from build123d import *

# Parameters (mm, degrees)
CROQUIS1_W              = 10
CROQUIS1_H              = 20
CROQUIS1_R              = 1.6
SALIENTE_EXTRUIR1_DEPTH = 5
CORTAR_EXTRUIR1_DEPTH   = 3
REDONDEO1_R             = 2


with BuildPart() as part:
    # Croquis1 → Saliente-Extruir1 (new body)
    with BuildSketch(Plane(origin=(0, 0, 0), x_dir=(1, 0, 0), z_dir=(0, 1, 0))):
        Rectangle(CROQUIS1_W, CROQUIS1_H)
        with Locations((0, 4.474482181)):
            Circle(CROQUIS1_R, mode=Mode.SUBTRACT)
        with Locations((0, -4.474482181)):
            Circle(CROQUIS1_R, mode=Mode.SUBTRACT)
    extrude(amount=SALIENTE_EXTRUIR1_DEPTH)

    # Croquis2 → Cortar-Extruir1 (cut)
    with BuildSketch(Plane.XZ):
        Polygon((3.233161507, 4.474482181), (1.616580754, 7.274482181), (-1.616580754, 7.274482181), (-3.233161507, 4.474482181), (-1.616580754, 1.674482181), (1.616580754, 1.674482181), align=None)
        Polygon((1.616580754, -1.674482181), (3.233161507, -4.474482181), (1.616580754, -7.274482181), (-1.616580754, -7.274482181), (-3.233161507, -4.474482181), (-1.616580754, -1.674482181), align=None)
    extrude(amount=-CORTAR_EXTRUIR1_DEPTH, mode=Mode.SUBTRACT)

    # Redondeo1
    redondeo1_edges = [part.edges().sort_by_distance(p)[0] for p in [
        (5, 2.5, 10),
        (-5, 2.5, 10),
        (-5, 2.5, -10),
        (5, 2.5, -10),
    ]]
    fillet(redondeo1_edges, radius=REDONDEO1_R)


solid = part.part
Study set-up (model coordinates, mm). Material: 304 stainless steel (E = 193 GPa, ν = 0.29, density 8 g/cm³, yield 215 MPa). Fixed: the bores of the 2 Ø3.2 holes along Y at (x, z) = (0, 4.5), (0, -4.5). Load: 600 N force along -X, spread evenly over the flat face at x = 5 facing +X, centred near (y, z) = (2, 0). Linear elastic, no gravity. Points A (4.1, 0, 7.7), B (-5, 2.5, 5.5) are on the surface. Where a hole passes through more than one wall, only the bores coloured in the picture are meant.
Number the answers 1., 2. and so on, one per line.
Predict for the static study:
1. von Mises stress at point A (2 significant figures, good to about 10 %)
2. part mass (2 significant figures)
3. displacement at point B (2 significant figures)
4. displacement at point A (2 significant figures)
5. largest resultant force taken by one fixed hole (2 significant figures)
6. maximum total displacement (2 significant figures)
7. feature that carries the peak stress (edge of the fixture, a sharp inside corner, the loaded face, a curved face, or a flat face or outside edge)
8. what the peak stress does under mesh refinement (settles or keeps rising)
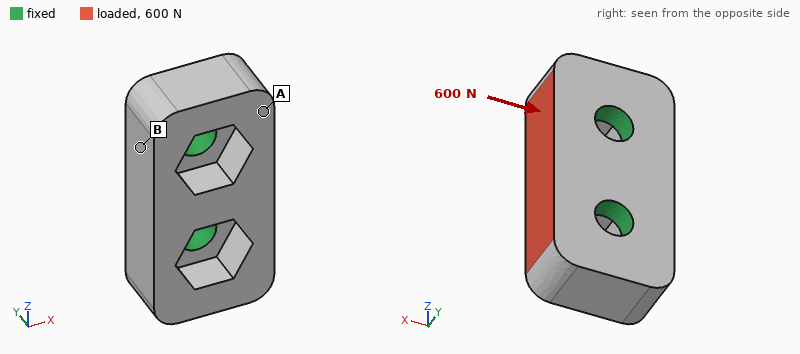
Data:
1. 12 MPa
2. 6.3 g
3. 0.92 µm
4. 1.5 µm
5. 300 N
6. 2.0 µm
7. edge of the fixture
8. keeps rising
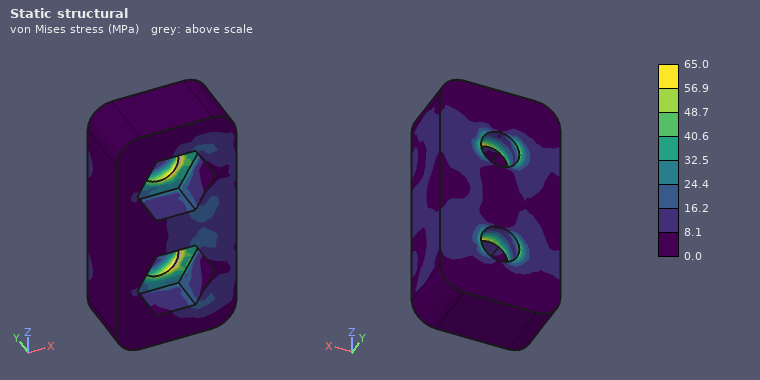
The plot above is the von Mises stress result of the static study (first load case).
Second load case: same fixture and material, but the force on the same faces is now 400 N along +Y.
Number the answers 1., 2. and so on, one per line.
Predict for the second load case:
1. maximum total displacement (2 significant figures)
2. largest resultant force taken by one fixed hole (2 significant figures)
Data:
1. 3.4 µm
2. 200 N
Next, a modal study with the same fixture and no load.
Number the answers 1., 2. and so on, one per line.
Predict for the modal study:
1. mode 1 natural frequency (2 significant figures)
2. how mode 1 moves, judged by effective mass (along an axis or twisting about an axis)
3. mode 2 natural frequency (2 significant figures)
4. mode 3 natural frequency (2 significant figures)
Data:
1. 39 kHz
2. along X
3. 51 kHz
4. 52 kHz
